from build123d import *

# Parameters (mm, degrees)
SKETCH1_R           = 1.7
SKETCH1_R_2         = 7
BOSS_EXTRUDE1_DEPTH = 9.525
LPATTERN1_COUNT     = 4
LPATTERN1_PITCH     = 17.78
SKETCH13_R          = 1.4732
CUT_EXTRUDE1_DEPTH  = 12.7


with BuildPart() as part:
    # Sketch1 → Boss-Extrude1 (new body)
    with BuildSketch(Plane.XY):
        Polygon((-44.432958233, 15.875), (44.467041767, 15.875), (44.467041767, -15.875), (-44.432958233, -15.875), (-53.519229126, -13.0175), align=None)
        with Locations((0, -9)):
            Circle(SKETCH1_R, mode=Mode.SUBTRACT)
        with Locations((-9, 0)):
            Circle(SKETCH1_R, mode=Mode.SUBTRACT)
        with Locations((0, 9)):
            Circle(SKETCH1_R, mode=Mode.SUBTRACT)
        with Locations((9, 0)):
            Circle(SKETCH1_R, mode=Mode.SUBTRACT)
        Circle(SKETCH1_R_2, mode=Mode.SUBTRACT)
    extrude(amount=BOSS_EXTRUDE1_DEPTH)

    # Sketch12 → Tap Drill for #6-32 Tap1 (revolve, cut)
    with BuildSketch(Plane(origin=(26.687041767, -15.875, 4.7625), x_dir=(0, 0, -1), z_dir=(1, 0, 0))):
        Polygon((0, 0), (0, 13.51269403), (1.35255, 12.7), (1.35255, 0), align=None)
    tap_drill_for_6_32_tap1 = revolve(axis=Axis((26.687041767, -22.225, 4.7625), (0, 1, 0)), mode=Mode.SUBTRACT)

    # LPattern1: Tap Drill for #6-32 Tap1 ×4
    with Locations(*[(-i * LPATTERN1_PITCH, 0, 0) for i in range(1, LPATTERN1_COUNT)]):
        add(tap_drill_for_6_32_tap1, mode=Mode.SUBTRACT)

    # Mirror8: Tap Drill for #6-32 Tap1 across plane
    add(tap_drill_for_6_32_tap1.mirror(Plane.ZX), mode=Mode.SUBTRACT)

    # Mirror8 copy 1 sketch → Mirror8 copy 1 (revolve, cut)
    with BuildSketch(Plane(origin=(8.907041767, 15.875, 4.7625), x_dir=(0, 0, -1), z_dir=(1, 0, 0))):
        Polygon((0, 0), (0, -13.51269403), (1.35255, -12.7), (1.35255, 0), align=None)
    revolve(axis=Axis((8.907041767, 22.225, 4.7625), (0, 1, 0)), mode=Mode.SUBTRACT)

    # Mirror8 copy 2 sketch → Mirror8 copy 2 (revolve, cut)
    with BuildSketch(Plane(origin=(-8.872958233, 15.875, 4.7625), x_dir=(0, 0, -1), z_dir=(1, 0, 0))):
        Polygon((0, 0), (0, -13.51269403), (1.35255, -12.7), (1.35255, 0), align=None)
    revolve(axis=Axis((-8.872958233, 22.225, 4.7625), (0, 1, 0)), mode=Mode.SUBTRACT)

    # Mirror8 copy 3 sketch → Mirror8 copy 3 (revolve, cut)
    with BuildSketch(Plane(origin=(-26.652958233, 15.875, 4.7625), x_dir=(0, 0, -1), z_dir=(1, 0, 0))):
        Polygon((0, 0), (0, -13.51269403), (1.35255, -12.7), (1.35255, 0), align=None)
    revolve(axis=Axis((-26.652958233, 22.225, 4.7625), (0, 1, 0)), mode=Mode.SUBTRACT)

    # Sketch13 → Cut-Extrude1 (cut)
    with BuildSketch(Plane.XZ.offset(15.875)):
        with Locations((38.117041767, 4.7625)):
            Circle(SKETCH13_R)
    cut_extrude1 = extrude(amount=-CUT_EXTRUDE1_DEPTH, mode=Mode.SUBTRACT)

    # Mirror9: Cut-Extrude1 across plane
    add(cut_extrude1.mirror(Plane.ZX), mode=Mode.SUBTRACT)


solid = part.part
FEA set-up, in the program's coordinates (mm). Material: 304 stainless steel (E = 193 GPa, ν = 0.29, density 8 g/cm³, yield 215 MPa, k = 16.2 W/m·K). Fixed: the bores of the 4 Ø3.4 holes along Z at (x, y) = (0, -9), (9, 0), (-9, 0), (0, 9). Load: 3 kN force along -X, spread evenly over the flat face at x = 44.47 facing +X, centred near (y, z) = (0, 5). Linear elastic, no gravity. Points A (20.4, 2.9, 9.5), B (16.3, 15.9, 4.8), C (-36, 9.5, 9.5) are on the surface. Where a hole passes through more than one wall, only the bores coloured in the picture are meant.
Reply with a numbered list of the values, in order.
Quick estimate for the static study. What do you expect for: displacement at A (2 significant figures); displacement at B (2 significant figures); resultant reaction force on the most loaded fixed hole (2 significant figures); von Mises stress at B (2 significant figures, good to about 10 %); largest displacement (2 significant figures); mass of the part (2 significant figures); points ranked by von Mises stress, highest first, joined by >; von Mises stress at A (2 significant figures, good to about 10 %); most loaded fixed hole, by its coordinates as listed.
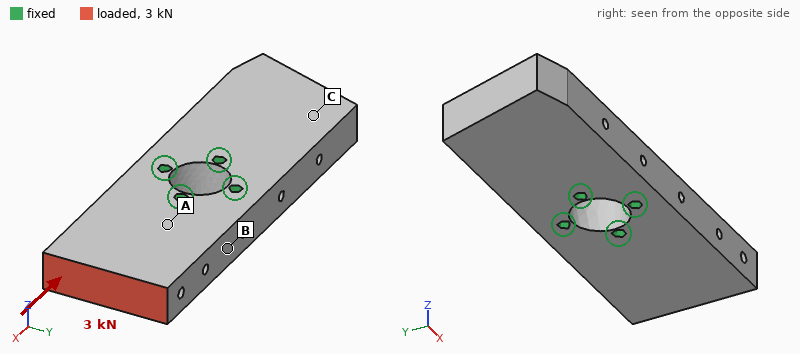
1. 0.88 µm
2. 0.87 µm
3. 1.5 kN
4. 6.6 MPa
5. 2.4 µm
6. 210 g
7. A > B > C
8. 13 MPa
9. (9, 0)
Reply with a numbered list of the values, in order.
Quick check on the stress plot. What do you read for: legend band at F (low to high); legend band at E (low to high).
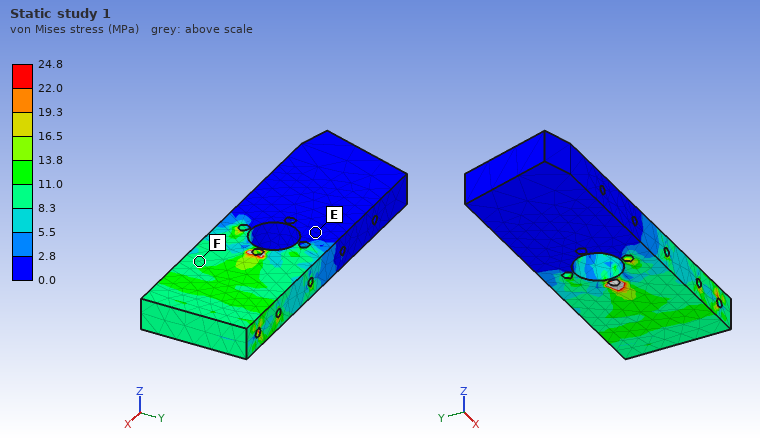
1. 8.3 to 11.0 MPa
2. 0.0 to 2.8 MPa
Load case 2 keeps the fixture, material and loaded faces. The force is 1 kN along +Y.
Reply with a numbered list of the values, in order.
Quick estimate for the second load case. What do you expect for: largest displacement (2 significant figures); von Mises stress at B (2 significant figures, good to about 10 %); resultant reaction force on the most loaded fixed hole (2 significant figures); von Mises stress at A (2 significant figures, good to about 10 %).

1. 9.5 µm
2. 18 MPa
3. 1.4 kN
4. 8.1 MPa
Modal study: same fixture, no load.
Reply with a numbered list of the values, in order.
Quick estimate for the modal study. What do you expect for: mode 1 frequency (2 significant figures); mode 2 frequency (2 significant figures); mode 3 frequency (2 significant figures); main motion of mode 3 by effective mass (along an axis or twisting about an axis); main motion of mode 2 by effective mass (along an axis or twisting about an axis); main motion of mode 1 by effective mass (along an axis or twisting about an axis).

1. 3900 Hz
2. 5100 Hz
3. 8300 Hz
4. along Y
5. along Z
6. along Z
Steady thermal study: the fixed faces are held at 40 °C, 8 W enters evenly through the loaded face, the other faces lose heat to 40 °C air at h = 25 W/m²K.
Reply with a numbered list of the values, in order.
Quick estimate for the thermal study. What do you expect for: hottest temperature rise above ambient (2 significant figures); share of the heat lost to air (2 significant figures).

1. 54 K
2. 31 %
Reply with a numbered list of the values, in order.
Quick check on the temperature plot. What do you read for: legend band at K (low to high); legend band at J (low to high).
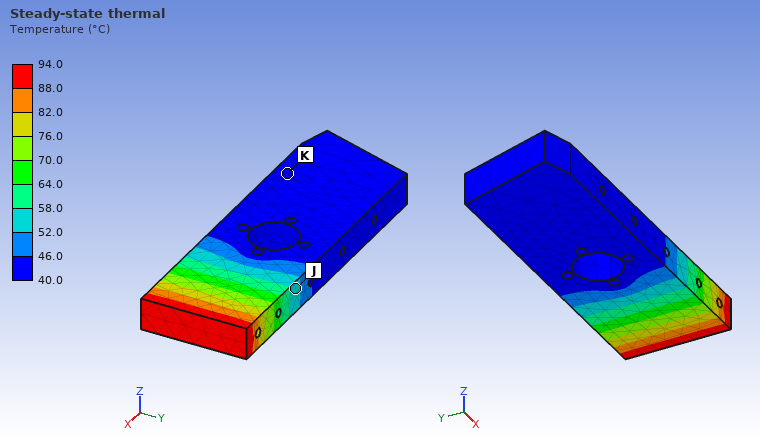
1. 40.0 to 46.0 °C
2. 52.0 to 58.0 °C
